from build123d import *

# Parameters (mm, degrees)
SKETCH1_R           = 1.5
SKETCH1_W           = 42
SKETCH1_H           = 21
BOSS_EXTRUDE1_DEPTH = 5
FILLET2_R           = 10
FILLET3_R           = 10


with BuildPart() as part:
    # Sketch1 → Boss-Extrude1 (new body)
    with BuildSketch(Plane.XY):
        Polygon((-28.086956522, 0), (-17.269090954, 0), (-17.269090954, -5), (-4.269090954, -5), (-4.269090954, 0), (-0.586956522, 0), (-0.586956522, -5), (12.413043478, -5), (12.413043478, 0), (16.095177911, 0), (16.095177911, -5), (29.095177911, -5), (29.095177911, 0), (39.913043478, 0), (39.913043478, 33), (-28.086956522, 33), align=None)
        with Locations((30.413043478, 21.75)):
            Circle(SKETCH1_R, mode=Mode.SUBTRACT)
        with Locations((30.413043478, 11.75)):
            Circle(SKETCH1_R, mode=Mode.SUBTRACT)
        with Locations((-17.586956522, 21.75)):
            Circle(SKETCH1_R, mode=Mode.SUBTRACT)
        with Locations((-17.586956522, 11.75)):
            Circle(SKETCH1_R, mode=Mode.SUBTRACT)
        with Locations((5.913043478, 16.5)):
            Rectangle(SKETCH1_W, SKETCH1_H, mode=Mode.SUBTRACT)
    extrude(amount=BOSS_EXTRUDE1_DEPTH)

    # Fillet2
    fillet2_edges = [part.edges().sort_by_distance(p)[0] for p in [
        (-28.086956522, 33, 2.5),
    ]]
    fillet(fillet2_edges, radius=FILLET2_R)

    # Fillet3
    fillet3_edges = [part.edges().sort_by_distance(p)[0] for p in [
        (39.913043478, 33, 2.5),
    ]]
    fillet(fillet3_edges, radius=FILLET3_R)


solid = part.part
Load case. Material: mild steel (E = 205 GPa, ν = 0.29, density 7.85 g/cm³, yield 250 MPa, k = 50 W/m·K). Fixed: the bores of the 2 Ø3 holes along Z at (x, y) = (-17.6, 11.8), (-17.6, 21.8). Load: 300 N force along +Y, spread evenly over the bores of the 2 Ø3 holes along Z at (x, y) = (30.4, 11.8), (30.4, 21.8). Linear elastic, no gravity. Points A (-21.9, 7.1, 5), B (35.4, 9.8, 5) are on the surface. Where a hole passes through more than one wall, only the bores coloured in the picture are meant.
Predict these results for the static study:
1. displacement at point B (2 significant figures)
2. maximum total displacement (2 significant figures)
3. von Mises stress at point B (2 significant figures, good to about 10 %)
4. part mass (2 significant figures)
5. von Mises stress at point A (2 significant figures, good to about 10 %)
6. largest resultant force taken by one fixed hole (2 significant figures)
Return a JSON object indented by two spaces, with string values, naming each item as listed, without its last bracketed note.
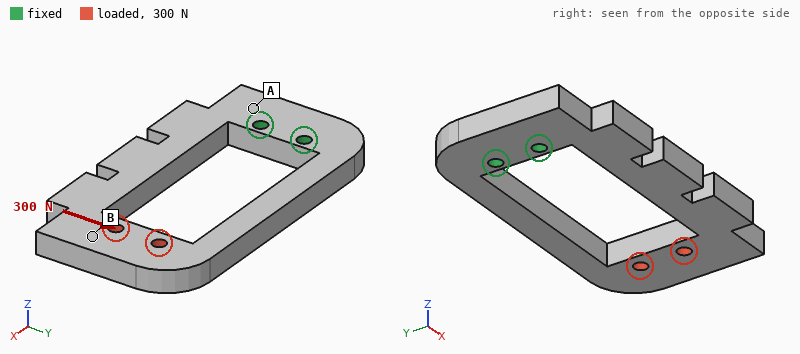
{
  "displacement at point B": "88 µm",
  "maximum total displacement": "91 µm",
  "von Mises stress at point B": "11 MPa",
  "part mass": "58 g",
  "von Mises stress at point A": "30 MPa",
  "largest resultant force taken by one fixed hole": "1.0 kN"
}
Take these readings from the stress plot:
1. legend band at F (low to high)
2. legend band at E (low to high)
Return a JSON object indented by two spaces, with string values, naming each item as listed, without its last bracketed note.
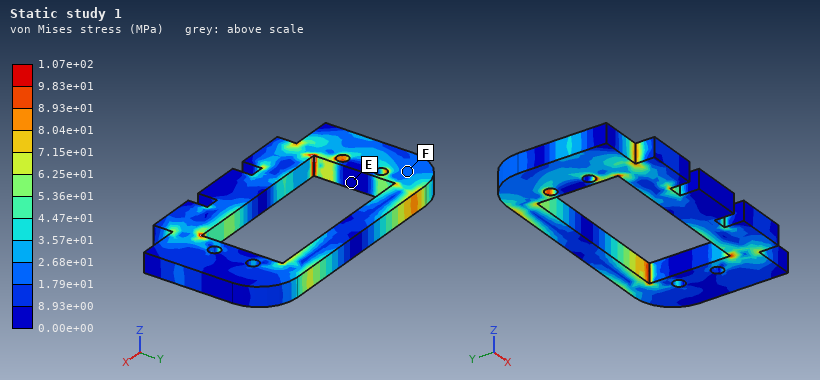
{
  "legend band at F": "1.79e+01 to 2.68e+01 MPa",
  "legend band at E": "0.00e+00 to 8.93e+00 MPa"
}
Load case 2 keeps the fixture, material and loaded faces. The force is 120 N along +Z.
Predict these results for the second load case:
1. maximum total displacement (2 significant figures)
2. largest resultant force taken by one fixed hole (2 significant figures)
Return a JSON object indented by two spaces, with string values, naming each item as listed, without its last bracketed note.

{
  "maximum total displacement": "0.26 mm",
  "largest resultant force taken by one fixed hole": "61 N"
}
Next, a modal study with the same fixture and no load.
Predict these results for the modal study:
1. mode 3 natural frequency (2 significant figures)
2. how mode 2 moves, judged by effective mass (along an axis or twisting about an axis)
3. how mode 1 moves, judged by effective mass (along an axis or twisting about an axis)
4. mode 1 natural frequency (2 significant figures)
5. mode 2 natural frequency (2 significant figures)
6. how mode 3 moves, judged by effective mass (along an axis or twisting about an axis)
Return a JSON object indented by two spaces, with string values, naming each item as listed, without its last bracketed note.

{
  "mode 3 natural frequency": "2400 Hz",
  "how mode 2 moves, judged by effective mass": "along Y",
  "how mode 1 moves, judged by effective mass": "along Z",
  "mode 1 natural frequency": "780 Hz",
  "mode 2 natural frequency": "1900 Hz",
  "how mode 3 moves, judged by effective mass": "twisting about X"
}
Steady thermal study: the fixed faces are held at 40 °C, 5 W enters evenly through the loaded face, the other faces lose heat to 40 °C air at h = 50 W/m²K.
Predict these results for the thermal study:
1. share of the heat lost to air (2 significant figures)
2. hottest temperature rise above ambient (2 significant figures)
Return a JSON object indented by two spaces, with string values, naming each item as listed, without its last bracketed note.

{
  "share of the heat lost to air": "72 %",
  "hottest temperature rise above ambient": "38 K"
}
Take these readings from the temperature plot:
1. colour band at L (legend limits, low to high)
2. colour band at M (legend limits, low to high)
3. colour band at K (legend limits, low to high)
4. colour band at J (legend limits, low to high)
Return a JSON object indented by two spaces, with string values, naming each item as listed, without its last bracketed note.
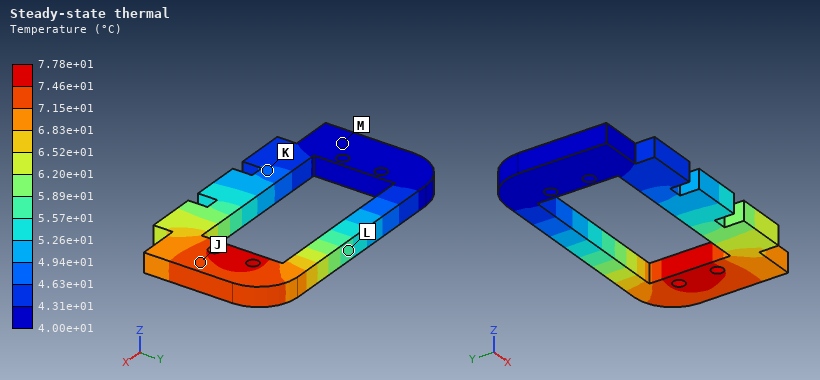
{
  "colour band at L": "5.57e+01 to 5.89e+01 °C",
  "colour band at M": "4.00e+01 to 4.31e+01 °C",
  "colour band at K": "4.63e+01 to 4.94e+01 °C",
  "colour band at J": "7.15e+01 to 7.46e+01 °C"
}
